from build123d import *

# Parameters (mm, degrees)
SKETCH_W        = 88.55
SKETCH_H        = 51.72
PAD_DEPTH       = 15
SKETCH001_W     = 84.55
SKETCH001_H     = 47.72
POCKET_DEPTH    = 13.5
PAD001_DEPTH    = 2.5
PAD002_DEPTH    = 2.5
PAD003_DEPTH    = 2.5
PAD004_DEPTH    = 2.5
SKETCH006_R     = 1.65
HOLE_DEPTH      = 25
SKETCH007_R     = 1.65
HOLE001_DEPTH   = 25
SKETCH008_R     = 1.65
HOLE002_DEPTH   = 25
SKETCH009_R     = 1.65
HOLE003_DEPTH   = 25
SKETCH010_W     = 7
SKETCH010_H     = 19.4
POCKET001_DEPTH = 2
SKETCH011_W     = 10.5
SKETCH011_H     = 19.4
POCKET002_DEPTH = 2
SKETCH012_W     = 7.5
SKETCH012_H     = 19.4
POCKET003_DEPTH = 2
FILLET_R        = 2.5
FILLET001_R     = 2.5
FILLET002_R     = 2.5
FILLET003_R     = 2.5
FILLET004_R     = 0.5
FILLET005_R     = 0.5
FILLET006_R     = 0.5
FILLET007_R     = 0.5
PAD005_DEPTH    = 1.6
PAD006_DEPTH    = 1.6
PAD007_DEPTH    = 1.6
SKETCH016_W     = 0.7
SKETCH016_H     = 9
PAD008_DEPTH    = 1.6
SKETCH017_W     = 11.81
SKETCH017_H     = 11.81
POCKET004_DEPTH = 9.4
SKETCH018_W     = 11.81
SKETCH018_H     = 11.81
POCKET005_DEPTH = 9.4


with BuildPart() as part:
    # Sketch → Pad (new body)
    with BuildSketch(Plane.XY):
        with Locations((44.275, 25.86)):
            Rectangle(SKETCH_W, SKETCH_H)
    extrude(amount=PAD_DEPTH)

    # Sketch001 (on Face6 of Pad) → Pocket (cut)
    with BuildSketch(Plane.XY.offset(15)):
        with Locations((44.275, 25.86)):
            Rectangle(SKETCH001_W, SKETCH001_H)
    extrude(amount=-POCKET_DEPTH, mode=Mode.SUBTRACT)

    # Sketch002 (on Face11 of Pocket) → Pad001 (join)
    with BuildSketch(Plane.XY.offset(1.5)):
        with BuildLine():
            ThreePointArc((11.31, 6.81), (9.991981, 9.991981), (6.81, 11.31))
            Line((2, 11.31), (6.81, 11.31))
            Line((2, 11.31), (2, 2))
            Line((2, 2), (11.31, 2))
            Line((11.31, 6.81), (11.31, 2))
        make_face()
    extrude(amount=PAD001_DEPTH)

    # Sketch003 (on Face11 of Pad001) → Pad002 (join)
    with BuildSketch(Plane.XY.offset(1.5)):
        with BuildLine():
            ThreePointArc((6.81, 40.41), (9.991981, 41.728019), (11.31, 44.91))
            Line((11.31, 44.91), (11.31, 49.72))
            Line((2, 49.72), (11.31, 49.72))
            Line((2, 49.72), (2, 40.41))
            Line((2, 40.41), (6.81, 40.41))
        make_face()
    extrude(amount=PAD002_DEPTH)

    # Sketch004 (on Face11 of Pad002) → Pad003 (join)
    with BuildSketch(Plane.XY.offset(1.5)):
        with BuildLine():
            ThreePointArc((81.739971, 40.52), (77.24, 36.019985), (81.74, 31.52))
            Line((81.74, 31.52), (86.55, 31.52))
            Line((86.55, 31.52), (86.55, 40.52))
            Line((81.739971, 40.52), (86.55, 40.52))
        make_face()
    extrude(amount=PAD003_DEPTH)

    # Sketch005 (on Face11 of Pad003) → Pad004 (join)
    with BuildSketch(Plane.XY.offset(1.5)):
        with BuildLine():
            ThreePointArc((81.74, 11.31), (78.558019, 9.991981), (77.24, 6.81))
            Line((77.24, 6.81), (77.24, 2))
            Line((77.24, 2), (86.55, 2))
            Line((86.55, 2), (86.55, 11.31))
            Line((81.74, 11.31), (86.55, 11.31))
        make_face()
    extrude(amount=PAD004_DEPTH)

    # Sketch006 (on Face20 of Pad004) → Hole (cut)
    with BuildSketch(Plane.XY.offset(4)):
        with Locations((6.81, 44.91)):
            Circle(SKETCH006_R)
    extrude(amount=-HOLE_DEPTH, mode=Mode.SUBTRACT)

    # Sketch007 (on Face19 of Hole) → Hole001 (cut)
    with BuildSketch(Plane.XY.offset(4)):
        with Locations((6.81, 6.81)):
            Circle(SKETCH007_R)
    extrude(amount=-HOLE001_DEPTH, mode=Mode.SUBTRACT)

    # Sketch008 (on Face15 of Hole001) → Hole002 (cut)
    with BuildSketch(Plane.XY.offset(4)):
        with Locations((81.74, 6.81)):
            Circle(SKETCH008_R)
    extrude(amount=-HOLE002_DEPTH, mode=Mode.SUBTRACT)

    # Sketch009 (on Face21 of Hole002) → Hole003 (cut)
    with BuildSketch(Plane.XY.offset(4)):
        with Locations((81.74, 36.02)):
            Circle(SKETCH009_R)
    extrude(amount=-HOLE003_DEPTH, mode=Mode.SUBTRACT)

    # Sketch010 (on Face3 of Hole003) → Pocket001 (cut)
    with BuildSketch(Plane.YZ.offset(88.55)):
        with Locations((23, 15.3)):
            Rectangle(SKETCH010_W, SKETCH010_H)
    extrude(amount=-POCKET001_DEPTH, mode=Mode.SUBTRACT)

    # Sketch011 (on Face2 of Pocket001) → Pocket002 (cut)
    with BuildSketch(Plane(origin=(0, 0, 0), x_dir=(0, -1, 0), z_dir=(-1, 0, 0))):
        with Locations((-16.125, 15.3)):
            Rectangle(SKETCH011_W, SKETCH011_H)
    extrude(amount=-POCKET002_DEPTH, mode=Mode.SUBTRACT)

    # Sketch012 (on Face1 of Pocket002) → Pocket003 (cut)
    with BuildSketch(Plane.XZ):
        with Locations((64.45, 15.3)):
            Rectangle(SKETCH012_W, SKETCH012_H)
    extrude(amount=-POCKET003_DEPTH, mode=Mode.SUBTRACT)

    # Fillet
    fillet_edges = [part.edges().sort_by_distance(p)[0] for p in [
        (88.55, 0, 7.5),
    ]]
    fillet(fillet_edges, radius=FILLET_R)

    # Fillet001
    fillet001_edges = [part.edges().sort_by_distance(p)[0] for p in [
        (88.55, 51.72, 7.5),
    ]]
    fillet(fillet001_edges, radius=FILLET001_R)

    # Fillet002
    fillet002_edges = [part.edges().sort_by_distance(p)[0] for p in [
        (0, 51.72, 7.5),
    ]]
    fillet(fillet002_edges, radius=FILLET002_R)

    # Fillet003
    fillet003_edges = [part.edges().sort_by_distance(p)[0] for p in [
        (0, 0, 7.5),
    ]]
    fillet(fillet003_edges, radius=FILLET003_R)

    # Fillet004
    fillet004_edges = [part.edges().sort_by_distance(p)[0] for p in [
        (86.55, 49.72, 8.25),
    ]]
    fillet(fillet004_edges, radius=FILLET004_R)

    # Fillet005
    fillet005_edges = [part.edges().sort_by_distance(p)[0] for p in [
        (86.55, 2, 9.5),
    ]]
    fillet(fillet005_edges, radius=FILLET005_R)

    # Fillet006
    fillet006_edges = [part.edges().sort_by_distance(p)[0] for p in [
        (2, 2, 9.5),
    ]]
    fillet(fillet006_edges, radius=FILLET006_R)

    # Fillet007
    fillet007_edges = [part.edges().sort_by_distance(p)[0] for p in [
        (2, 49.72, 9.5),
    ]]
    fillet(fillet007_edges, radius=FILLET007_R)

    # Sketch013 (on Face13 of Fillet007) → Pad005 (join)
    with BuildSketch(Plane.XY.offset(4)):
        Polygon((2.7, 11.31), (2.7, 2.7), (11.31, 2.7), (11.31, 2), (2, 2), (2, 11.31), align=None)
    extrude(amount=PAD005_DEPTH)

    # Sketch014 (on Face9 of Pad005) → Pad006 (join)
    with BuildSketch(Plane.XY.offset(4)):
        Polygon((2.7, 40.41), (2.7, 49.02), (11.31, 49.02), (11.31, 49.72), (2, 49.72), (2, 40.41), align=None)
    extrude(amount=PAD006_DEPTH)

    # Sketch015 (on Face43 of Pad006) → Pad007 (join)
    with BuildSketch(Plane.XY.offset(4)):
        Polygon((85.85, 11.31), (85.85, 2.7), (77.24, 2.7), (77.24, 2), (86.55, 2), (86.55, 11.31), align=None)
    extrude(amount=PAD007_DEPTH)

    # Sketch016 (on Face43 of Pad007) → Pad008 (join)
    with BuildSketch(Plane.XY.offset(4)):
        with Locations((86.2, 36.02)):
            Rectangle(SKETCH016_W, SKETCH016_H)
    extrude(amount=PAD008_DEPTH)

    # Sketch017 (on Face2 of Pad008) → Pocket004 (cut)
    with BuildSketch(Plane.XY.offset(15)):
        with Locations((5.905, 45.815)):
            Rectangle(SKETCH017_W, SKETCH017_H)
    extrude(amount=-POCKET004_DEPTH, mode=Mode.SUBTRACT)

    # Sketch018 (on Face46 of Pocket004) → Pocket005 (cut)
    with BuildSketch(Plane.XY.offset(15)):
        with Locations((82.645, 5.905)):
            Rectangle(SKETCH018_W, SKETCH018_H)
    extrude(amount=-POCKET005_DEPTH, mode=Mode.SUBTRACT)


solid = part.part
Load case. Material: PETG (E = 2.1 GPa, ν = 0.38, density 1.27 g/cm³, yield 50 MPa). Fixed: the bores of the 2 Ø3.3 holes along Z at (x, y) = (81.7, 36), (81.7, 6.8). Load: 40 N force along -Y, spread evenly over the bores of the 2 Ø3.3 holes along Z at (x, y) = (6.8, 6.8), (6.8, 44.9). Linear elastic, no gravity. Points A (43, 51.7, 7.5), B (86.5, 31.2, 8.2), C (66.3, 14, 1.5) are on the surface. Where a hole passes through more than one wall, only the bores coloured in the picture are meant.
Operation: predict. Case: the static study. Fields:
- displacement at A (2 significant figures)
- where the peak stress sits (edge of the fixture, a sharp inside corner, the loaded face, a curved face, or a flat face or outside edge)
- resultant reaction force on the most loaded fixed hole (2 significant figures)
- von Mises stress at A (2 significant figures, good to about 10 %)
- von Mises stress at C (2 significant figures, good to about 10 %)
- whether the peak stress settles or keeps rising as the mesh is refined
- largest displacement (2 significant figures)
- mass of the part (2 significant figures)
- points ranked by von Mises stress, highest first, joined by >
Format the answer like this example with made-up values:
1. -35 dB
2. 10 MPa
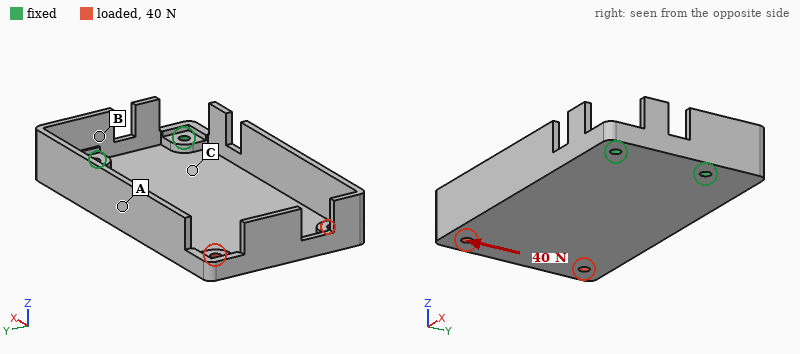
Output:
1. 0.30 mm
2. edge of the fixture
3. 96 N
4. 1.1 MPa
5. 2.6 MPa
6. keeps rising
7. 1.2 mm
8. 17 g
9. C > A > B
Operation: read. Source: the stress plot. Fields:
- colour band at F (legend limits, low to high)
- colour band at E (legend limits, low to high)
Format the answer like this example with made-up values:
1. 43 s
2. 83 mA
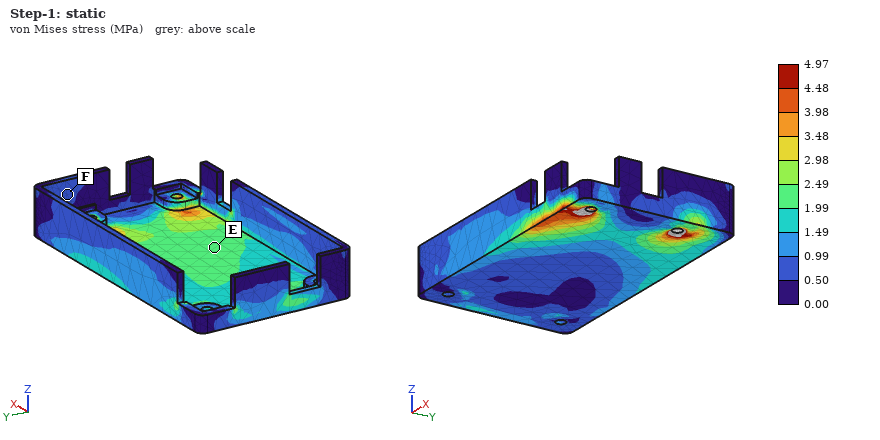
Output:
1. 0.50 to 0.99 MPa
2. 1.99 to 2.49 MPa
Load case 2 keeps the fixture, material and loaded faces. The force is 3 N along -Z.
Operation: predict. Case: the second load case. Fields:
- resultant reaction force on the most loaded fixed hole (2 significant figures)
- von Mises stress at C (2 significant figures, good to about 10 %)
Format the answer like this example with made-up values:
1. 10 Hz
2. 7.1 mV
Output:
1. 2.8 N
2. 0.53 MPa
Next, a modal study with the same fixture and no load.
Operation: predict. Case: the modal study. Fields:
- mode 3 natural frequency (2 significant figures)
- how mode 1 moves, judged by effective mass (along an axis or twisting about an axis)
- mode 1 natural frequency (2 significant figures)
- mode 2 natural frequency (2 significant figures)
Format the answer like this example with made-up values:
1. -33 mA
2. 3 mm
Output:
1. 670 Hz
2. along Z
3. 100 Hz
4. 180 Hz
